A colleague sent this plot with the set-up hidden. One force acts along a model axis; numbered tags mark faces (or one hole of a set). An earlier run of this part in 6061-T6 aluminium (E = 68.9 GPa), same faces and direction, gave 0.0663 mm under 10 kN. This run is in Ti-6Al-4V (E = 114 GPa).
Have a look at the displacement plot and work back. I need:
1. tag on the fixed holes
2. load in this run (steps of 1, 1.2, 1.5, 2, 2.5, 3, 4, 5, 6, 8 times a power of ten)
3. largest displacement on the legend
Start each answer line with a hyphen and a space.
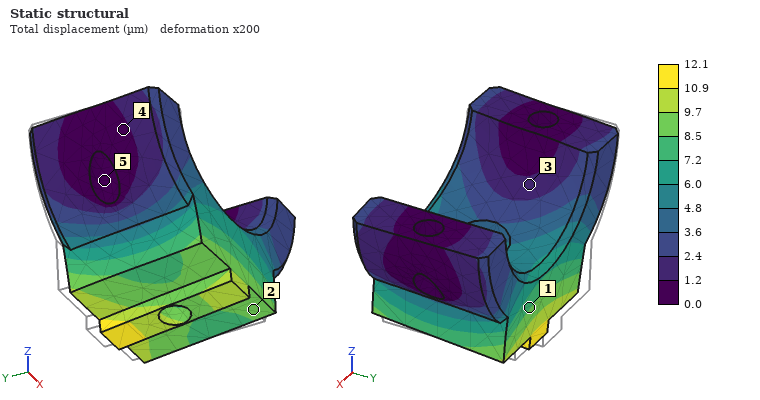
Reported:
- 5
- 3 kN
- 12.1 µm
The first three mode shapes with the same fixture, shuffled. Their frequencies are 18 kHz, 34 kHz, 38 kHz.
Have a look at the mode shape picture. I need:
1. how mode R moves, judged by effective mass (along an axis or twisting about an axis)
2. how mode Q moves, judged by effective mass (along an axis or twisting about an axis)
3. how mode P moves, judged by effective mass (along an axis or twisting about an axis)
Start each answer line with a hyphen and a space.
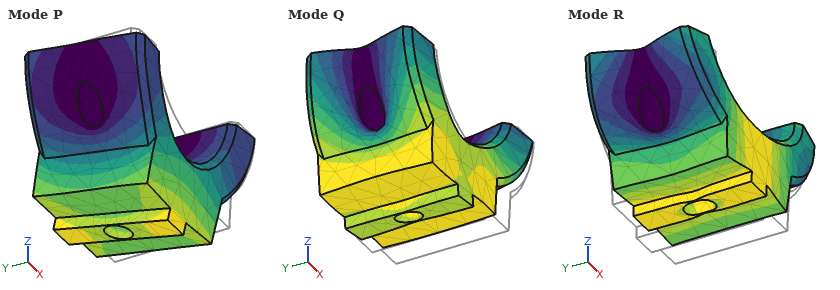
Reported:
- along Z
- along X
- along Y
